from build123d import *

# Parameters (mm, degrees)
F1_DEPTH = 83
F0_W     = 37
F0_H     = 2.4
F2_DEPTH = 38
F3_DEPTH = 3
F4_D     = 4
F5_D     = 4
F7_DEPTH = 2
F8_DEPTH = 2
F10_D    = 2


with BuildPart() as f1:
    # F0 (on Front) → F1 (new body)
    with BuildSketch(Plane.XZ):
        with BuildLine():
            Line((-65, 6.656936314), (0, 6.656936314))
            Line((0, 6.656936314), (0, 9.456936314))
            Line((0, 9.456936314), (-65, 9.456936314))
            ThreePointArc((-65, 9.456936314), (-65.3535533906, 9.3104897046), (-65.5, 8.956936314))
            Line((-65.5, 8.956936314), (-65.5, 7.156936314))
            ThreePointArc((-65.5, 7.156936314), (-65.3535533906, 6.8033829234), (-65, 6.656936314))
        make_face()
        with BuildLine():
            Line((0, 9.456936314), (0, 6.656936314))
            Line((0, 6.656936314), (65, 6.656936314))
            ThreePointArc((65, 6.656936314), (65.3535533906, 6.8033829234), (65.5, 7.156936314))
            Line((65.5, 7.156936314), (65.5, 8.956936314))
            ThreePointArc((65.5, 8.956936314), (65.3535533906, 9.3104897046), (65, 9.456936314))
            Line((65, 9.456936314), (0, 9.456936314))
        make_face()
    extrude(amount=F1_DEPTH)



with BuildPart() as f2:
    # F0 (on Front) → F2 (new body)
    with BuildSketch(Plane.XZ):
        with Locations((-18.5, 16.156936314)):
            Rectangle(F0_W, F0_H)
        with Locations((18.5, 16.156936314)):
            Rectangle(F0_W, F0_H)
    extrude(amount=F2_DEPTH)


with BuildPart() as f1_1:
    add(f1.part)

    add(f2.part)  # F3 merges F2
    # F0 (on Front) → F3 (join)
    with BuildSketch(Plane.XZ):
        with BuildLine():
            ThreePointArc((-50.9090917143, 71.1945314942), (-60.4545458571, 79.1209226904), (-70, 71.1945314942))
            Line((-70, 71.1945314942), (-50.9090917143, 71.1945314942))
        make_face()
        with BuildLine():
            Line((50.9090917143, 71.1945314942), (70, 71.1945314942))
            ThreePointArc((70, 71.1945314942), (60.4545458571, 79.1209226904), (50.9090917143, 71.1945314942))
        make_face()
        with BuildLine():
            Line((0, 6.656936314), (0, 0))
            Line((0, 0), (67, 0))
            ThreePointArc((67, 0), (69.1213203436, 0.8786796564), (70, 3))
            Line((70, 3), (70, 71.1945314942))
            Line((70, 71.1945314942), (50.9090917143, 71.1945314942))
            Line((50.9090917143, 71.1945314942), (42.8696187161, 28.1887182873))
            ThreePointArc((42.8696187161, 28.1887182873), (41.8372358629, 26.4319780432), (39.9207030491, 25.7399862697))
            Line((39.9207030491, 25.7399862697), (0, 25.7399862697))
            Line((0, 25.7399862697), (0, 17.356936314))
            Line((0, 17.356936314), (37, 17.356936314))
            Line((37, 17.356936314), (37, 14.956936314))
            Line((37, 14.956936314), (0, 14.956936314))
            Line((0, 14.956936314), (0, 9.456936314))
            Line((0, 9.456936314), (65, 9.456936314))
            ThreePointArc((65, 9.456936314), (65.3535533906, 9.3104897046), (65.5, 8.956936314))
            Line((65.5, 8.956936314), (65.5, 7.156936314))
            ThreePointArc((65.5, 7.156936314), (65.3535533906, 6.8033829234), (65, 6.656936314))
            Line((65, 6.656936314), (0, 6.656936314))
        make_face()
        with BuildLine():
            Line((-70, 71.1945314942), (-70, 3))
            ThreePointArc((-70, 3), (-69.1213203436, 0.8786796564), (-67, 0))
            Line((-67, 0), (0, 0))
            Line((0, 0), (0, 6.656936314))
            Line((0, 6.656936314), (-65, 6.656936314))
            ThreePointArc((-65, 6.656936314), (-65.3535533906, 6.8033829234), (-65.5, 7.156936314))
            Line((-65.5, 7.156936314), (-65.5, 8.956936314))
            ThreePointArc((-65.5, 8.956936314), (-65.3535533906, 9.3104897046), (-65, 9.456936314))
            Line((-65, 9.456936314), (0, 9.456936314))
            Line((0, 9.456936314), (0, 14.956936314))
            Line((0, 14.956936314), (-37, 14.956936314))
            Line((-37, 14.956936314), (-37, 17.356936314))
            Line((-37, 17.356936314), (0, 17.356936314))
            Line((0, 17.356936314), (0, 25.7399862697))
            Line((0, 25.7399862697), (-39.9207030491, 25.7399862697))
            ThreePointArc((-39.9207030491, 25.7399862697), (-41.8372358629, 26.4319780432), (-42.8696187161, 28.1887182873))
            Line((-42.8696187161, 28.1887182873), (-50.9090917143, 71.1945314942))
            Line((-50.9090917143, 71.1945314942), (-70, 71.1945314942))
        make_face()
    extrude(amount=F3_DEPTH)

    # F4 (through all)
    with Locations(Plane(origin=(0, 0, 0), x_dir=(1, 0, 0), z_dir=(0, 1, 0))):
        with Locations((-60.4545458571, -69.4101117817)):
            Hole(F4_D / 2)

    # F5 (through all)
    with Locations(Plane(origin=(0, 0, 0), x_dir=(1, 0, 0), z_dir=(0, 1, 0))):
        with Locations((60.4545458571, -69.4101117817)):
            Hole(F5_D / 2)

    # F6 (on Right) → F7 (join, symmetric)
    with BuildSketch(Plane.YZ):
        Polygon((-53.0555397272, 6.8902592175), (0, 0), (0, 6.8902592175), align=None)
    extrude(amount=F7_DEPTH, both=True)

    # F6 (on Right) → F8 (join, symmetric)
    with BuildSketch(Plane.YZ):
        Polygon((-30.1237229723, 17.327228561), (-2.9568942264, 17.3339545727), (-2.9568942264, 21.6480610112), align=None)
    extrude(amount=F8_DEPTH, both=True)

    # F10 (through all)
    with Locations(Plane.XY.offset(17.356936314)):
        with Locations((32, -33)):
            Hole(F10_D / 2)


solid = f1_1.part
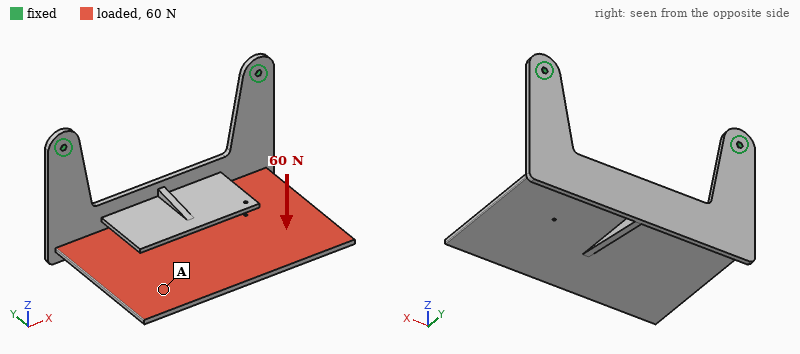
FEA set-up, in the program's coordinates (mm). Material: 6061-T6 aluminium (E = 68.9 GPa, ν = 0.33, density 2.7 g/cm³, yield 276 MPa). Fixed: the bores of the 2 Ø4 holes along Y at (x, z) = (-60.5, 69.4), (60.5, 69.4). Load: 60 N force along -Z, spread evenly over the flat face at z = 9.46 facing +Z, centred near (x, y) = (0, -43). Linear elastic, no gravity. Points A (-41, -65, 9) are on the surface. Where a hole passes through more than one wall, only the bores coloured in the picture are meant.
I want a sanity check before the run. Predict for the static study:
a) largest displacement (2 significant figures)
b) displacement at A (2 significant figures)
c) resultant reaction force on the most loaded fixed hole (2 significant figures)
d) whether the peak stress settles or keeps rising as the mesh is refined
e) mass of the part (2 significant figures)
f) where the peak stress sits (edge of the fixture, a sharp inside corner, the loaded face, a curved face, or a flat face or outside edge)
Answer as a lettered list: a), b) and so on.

a) 1.8 mm
b) 1.4 mm
c) 33 N
d) keeps rising
e) 150 g
f) edge of the fixture
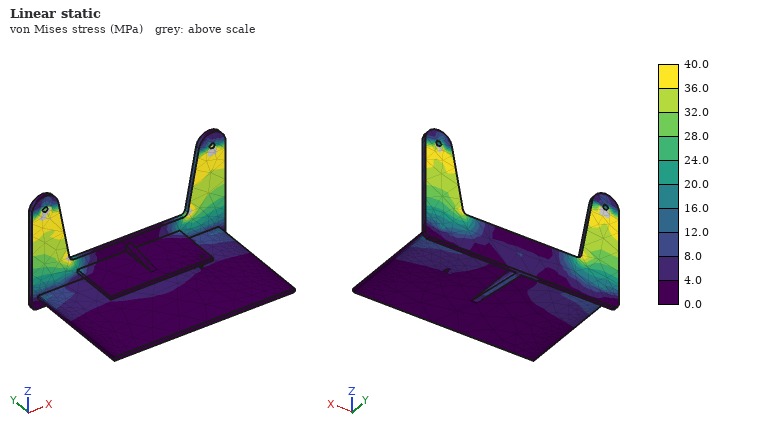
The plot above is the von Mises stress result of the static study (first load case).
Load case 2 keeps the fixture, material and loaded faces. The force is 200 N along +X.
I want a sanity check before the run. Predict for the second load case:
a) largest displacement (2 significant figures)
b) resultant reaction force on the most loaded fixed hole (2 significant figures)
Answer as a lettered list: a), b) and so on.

a) 0.86 mm
b) 140 N
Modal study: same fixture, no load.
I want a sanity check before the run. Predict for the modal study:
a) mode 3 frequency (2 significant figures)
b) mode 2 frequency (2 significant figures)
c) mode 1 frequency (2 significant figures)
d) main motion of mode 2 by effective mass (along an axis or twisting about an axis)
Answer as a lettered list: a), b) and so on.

a) 330 Hz
b) 270 Hz
c) 99 Hz
d) along X
